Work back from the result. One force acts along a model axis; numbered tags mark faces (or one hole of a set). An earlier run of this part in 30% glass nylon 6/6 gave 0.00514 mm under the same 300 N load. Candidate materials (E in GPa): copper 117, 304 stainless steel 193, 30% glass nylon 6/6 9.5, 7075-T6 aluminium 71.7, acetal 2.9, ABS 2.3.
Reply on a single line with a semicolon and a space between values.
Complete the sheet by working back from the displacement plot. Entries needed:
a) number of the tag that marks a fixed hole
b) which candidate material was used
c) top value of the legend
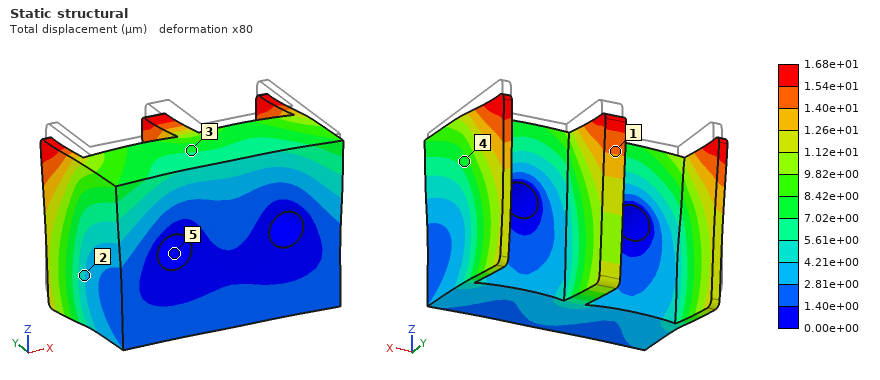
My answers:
5; acetal; 1.68e+01 µm
